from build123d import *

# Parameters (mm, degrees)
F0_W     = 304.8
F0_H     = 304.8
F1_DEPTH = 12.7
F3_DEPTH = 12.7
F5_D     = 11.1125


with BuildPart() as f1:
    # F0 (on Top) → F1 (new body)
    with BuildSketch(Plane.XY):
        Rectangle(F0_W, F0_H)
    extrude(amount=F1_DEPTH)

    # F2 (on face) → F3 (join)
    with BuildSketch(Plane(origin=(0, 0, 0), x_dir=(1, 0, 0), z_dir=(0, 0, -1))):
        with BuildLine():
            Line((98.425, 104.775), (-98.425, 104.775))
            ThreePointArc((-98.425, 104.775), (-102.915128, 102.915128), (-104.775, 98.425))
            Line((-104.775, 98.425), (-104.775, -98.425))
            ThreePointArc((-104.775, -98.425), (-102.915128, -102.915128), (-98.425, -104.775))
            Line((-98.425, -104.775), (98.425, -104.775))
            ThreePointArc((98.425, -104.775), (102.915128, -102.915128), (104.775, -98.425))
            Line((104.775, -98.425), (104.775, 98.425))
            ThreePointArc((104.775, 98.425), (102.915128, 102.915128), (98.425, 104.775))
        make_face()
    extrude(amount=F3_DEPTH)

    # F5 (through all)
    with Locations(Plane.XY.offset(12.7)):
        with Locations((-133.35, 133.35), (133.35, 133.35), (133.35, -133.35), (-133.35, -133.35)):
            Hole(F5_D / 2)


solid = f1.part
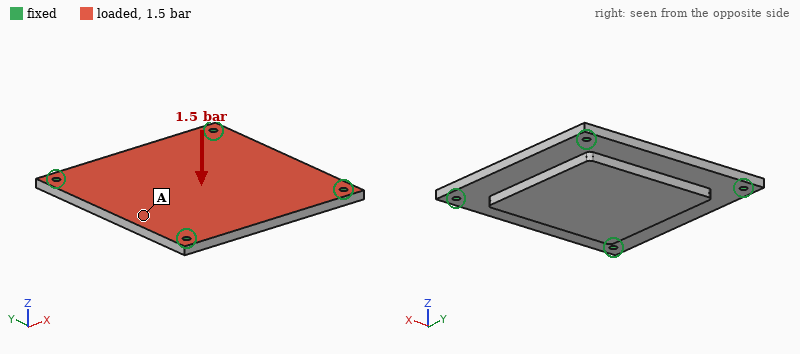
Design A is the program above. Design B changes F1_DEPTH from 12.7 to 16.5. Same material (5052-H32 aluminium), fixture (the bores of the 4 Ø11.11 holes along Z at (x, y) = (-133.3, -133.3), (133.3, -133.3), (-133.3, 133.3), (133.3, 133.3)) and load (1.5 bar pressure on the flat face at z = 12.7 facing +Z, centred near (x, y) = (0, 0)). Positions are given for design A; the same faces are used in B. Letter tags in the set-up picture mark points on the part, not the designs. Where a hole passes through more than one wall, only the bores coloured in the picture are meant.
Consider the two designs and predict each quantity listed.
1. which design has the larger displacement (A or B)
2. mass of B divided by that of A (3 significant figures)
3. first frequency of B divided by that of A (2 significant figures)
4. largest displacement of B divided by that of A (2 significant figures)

A
1.20
1.2
0.60
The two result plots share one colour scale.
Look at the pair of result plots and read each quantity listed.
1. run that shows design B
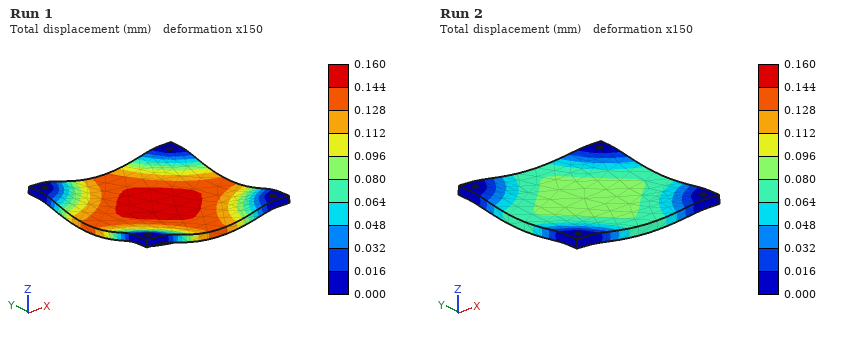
Run 2
